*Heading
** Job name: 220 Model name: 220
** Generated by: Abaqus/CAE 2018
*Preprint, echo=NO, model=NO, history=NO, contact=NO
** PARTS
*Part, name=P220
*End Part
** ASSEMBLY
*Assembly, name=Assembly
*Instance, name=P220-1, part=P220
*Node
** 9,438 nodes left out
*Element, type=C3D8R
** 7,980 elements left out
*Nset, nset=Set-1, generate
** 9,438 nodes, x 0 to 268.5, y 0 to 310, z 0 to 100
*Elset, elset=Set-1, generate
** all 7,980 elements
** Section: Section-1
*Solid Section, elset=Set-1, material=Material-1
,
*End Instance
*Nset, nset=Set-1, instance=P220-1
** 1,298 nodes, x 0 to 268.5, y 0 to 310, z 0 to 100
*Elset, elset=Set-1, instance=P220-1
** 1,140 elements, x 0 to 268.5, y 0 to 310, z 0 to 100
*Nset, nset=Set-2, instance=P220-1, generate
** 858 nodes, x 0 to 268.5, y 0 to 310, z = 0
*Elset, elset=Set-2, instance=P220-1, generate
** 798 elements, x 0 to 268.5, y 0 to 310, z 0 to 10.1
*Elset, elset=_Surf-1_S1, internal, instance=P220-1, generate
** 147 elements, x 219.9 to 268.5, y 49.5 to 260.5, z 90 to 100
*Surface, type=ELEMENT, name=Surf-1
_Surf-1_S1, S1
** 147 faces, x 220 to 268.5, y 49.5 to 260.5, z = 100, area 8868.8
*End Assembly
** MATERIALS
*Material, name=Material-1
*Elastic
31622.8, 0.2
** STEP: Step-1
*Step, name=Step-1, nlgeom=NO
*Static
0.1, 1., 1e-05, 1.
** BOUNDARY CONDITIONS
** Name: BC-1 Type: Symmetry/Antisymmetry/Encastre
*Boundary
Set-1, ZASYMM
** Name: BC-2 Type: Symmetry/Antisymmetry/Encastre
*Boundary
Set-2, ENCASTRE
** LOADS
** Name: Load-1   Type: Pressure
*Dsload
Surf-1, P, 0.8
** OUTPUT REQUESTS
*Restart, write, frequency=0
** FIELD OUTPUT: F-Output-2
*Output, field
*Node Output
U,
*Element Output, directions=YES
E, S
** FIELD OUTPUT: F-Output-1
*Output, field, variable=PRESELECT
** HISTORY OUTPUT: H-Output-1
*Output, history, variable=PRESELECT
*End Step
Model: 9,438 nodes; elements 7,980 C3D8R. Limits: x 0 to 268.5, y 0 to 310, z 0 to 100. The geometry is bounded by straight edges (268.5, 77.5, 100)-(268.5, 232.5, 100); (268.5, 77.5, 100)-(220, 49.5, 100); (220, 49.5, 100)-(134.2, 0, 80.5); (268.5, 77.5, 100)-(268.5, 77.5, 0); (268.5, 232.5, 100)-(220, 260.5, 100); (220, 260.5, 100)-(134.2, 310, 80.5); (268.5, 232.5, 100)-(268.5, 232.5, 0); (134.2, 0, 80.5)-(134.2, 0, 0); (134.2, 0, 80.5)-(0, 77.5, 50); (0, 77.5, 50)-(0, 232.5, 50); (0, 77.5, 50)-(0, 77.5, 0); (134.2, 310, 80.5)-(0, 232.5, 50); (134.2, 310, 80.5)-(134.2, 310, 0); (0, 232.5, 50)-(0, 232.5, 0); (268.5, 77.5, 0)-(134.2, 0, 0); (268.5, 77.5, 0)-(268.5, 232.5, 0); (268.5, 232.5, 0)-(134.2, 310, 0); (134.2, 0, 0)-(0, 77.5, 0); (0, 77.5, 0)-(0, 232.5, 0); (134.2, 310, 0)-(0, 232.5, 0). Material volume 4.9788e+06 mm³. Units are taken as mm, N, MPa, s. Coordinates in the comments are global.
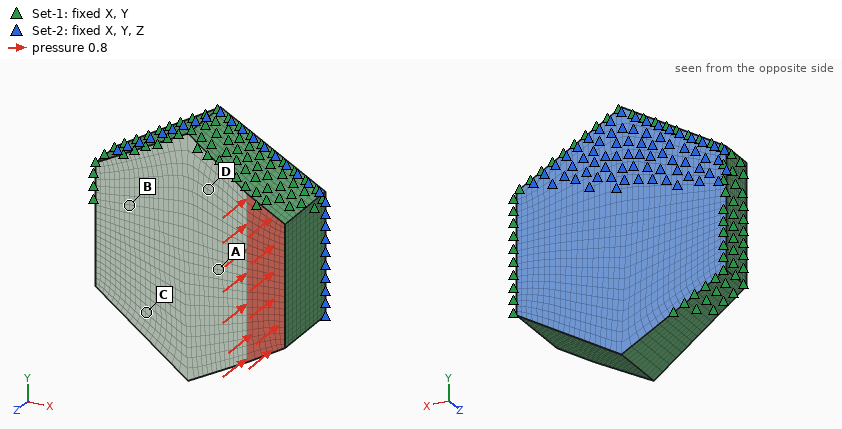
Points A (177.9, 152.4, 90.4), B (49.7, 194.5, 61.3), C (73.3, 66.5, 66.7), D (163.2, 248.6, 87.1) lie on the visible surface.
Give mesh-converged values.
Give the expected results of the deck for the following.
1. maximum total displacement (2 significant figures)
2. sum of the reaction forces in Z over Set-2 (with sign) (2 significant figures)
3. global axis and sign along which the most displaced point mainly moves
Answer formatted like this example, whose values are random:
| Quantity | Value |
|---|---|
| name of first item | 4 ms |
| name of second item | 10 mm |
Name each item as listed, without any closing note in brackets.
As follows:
| Quantity | Value |
|---|---|
| maximum total displacement | 0.0020 mm |
| sum of the reaction forces in Z over Set-2 (with sign) | 7100 N |
| global axis and sign along which the most displaced point mainly moves | -Z |
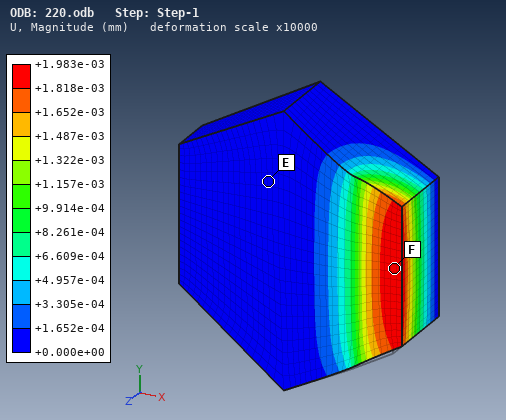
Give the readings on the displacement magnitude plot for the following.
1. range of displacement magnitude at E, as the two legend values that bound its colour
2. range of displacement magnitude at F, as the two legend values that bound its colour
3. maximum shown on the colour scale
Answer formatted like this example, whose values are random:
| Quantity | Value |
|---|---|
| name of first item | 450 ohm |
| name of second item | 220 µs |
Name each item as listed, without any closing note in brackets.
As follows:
| Quantity | Value |
|---|---|
| range of displacement magnitude at E, as the two legend values that bound its colour | +0.000e+00 to +1.652e-04 mm |
| range of displacement magnitude at F, as the two legend values that bound its colour | +1.818e-03 to +1.983e-03 mm |
| maximum shown on the colour scale | +1.983e-03 mm |
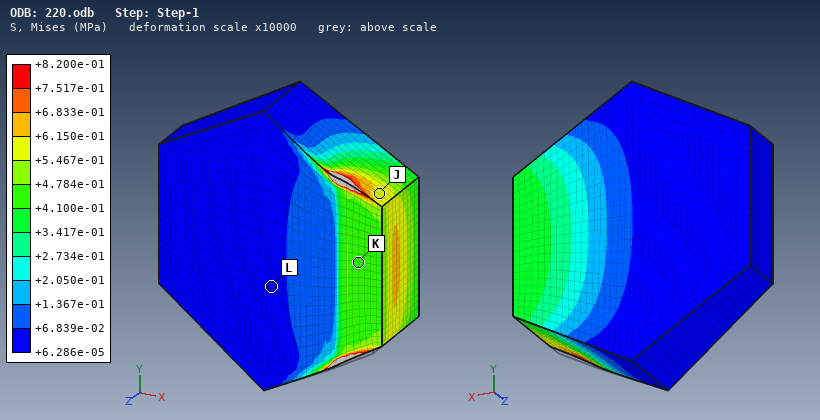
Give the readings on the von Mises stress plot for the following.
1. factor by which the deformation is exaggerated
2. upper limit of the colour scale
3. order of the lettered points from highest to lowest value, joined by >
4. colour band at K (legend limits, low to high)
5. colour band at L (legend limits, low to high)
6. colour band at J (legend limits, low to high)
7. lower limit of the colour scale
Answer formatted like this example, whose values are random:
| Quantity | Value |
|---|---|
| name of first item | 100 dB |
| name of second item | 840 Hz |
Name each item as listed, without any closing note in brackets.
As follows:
| Quantity | Value |
|---|---|
| factor by which the deformation is exaggerated | 10000 |
| upper limit of the colour scale | +8.200e-01 MPa |
| order of the lettered points from highest to lowest value, joined by > | J > K > L |
| colour band at K | +4.100e-01 to +4.784e-01 MPa |
| colour band at L | +6.286e-05 to +6.839e-02 MPa |
| colour band at J | +5.467e-01 to +6.150e-01 MPa |
| lower limit of the colour scale | +6.286e-05 MPa |
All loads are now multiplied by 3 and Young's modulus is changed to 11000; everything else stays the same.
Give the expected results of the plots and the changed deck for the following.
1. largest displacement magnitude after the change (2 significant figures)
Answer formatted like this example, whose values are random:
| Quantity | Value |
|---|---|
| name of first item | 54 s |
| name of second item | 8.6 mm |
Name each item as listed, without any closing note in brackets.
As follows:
| Quantity | Value |
|---|---|
| largest displacement magnitude after the change | 0.017 mm |
